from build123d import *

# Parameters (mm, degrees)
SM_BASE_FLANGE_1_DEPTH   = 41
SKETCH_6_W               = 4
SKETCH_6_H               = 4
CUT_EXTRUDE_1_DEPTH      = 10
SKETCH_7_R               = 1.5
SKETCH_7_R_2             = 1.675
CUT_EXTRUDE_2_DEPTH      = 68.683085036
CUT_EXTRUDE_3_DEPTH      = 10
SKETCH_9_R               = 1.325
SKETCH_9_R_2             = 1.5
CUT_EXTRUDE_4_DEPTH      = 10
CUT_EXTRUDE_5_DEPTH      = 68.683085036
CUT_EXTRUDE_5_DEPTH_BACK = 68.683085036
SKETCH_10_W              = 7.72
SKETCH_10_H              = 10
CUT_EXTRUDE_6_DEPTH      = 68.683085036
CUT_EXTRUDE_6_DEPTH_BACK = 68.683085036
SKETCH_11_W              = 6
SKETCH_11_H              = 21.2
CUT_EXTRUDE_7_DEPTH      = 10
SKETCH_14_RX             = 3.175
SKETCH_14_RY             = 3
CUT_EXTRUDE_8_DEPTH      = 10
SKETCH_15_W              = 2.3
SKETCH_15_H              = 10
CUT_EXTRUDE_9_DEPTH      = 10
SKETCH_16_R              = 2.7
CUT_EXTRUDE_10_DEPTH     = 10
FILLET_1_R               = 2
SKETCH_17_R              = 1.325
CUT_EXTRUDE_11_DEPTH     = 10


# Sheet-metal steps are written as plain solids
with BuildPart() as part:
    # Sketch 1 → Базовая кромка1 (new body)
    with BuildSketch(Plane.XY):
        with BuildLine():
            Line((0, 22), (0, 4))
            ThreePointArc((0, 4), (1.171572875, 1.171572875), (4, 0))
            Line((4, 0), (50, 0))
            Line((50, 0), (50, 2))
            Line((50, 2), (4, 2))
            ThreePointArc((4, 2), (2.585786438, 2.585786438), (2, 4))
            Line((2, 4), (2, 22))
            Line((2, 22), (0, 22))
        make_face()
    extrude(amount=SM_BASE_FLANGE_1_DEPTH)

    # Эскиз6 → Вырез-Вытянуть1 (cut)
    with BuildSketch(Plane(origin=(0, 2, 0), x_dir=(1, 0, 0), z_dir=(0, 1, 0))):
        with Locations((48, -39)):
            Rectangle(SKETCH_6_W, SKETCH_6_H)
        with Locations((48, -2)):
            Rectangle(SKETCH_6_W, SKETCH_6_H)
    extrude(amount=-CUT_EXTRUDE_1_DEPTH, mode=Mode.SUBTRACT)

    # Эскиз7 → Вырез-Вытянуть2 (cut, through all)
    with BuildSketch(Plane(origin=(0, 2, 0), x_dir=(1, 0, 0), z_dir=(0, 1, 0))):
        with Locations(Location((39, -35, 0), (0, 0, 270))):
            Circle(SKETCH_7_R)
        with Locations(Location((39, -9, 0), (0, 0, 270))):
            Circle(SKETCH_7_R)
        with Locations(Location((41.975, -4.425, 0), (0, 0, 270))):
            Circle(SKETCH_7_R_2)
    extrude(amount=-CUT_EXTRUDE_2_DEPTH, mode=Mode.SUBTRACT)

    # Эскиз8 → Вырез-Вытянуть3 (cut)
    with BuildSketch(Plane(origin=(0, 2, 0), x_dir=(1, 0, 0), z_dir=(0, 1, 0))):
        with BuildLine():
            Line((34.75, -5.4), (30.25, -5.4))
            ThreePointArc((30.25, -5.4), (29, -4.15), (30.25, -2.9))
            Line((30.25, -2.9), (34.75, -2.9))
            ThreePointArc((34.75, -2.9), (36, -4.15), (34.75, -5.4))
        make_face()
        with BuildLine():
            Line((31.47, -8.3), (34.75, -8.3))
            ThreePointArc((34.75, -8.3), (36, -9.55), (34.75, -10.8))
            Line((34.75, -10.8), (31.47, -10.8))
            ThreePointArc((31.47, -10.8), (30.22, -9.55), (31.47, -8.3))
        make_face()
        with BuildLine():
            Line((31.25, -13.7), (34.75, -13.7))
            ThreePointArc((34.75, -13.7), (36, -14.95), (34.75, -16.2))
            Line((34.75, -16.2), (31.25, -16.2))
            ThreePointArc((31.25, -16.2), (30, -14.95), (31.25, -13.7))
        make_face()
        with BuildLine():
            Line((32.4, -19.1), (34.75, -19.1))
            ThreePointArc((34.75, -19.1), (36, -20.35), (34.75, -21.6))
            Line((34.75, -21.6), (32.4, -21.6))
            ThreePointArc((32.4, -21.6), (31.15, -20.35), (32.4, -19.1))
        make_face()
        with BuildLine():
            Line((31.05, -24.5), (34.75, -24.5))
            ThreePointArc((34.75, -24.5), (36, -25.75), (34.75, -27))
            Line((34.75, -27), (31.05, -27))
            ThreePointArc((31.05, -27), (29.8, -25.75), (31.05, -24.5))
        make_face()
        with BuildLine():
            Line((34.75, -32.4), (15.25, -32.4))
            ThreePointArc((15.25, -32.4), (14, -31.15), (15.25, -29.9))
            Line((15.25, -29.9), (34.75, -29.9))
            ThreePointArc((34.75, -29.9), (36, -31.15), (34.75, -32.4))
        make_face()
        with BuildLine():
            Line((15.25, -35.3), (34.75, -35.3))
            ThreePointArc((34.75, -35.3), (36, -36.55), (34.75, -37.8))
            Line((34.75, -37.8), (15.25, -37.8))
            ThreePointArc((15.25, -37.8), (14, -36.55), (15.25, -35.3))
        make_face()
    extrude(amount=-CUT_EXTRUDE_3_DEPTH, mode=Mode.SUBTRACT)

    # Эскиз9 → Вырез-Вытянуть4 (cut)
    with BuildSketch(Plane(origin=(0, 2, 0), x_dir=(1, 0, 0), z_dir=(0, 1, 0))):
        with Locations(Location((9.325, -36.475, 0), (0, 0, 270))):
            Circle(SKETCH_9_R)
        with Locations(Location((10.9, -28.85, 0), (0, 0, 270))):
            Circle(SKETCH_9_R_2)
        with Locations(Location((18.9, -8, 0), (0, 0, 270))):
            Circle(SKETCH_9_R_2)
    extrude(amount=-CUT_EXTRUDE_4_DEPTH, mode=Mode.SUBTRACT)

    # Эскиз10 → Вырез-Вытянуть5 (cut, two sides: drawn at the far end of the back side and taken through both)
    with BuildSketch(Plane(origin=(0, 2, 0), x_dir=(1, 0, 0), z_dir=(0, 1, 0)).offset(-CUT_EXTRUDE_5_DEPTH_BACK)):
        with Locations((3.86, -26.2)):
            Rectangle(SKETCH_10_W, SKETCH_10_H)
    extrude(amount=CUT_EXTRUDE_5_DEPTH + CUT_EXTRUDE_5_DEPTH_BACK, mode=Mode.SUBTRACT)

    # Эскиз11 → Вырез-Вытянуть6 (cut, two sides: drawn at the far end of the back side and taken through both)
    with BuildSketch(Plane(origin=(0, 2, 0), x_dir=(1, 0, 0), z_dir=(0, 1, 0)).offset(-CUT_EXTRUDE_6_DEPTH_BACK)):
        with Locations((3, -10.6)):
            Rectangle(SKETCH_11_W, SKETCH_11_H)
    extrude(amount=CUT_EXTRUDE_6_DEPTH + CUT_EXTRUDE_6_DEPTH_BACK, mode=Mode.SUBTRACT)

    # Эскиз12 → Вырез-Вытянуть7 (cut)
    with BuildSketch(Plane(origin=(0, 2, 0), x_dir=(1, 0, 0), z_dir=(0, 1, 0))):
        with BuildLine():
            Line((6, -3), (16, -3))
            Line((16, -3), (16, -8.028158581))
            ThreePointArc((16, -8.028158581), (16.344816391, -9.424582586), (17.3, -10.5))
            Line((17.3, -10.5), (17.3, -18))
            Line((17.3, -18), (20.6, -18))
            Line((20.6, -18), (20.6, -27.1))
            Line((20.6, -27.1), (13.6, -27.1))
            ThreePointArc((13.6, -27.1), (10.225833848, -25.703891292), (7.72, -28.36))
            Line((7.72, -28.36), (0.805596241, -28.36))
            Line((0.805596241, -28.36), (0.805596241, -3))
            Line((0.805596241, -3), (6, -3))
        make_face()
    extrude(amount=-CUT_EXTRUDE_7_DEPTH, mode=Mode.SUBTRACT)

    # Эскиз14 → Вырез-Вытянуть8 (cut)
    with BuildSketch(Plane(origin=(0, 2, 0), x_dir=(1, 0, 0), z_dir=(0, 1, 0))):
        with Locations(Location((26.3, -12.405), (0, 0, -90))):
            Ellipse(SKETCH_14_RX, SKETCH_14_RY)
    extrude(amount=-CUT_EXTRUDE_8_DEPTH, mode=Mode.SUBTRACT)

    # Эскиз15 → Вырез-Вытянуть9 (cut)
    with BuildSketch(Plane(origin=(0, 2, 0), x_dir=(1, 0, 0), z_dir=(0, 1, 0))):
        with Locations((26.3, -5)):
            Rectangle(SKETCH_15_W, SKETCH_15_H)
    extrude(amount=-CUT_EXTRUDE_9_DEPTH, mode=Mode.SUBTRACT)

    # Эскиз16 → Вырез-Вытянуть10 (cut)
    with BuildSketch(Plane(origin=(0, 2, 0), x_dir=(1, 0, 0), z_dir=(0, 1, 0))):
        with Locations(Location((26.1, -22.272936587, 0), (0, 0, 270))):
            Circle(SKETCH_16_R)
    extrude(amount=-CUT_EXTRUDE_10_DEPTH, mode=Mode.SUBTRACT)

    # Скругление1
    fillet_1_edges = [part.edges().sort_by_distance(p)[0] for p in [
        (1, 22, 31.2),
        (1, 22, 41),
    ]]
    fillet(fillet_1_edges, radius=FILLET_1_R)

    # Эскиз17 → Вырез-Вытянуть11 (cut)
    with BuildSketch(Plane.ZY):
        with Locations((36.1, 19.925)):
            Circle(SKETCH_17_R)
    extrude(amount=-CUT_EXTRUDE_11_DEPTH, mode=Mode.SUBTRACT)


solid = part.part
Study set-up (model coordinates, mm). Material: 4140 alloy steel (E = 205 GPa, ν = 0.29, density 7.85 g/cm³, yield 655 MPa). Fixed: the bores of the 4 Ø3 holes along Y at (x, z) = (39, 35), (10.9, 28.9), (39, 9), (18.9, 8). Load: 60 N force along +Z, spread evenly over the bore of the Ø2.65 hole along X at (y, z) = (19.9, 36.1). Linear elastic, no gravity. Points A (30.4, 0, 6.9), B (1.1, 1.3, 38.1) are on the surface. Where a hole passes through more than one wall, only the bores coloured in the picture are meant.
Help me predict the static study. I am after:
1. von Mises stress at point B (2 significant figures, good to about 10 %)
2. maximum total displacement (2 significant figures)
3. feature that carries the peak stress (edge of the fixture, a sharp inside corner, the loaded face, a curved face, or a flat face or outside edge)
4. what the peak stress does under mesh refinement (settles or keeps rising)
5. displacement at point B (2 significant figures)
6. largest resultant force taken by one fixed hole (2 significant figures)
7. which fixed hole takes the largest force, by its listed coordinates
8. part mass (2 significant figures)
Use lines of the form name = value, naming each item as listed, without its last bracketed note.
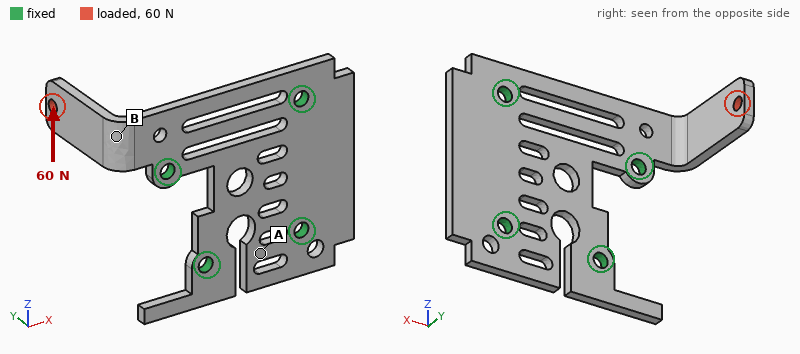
von Mises stress at point B = 77 MPa
maximum total displacement = 0.21 mm
feature that carries the peak stress = edge of the fixture
what the peak stress does under mesh refinement = keeps rising
displacement at point B = 0.051 mm
largest resultant force taken by one fixed hole = 80 N
which fixed hole takes the largest force, by its listed coordinates = (10.9, 28.9)
part mass = 22 g
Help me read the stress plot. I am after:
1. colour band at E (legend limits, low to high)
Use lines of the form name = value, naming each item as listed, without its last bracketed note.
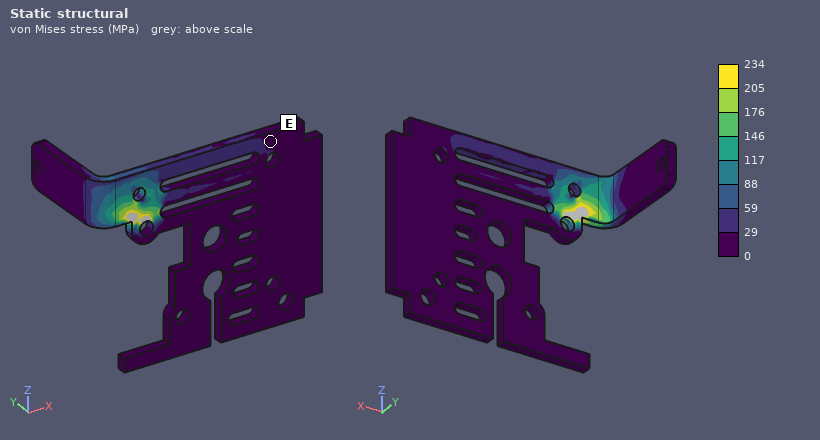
colour band at E = 0 to 29 MPa
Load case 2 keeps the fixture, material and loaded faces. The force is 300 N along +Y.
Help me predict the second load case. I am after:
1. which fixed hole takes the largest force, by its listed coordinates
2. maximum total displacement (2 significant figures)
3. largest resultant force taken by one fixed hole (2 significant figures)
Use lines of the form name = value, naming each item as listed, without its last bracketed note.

which fixed hole takes the largest force, by its listed coordinates = (10.9, 28.9)
maximum total displacement = 0.44 mm
largest resultant force taken by one fixed hole = 340 N
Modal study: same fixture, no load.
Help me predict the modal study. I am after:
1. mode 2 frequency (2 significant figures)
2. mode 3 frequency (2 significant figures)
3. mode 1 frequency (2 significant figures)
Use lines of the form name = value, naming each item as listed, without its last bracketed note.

mode 2 frequency = 2600 Hz
mode 3 frequency = 6900 Hz
mode 1 frequency = 2000 Hz
